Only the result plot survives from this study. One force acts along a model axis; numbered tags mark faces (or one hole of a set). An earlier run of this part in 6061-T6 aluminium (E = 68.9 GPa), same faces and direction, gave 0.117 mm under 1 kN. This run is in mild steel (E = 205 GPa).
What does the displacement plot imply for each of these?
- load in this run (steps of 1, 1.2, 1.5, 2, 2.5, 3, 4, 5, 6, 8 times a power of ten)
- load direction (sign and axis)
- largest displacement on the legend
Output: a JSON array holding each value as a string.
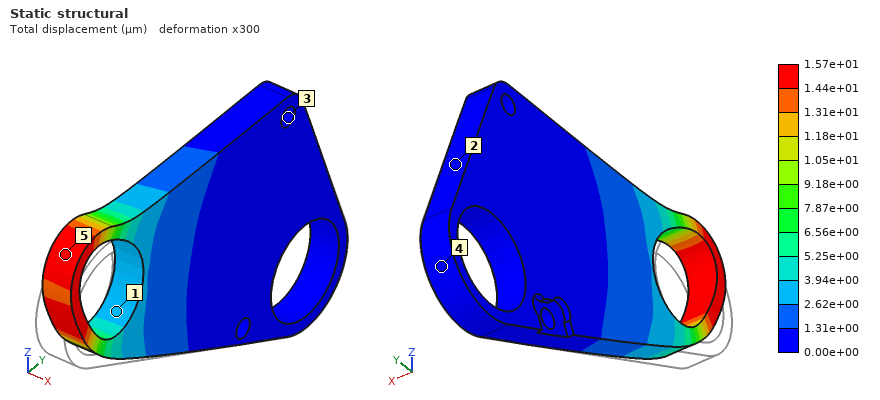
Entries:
["400 N", "+Z", "1.57e+01 µm"]
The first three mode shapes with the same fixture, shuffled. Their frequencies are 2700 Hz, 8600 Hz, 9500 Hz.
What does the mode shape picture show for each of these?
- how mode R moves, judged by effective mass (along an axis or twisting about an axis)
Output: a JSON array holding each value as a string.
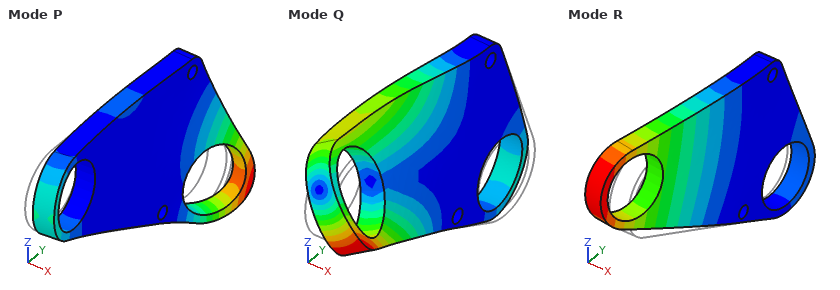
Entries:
["along X"]
